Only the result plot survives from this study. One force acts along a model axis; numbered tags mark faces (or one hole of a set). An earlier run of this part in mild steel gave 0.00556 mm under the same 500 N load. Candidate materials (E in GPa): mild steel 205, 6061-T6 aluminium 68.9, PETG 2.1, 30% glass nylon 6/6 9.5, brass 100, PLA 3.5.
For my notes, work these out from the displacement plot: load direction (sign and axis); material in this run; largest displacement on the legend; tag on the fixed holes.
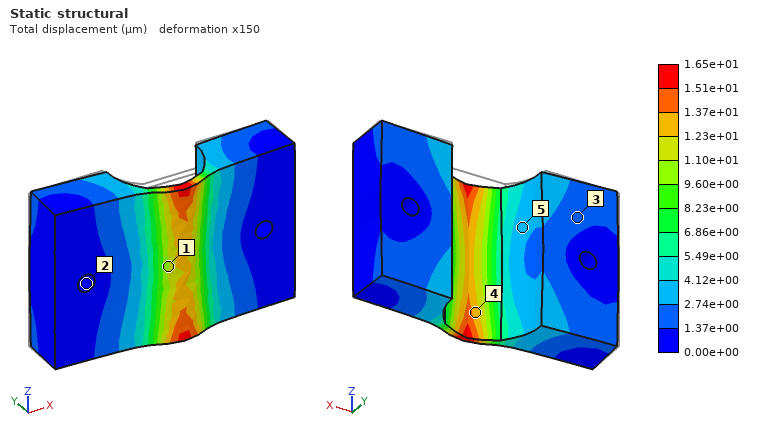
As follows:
-Y
6061-T6 aluminium
1.65e+01 µm
2
